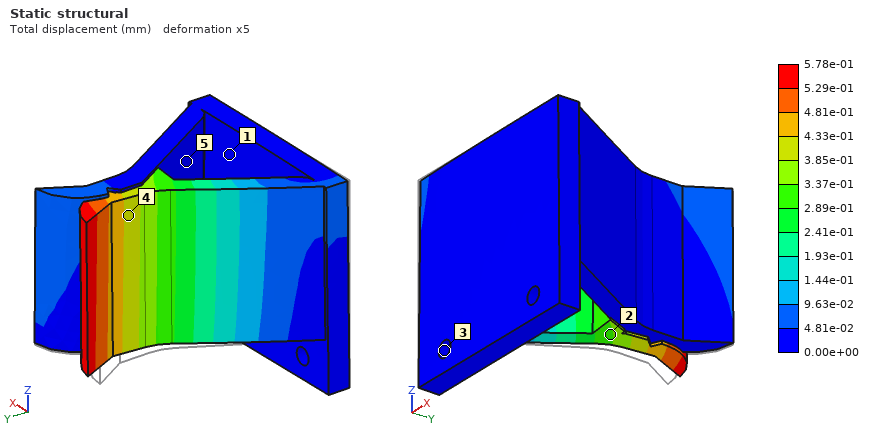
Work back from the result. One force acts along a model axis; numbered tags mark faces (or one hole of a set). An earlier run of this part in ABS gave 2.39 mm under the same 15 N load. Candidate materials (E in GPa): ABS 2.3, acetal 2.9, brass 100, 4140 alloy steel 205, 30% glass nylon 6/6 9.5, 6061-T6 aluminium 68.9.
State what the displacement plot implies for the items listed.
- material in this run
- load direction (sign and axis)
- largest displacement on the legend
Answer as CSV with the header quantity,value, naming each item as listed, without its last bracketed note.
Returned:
quantity,value
material in this run,30% glass nylon 6/6
load direction,+X
largest displacement on the legend,5.78e-01 mm
